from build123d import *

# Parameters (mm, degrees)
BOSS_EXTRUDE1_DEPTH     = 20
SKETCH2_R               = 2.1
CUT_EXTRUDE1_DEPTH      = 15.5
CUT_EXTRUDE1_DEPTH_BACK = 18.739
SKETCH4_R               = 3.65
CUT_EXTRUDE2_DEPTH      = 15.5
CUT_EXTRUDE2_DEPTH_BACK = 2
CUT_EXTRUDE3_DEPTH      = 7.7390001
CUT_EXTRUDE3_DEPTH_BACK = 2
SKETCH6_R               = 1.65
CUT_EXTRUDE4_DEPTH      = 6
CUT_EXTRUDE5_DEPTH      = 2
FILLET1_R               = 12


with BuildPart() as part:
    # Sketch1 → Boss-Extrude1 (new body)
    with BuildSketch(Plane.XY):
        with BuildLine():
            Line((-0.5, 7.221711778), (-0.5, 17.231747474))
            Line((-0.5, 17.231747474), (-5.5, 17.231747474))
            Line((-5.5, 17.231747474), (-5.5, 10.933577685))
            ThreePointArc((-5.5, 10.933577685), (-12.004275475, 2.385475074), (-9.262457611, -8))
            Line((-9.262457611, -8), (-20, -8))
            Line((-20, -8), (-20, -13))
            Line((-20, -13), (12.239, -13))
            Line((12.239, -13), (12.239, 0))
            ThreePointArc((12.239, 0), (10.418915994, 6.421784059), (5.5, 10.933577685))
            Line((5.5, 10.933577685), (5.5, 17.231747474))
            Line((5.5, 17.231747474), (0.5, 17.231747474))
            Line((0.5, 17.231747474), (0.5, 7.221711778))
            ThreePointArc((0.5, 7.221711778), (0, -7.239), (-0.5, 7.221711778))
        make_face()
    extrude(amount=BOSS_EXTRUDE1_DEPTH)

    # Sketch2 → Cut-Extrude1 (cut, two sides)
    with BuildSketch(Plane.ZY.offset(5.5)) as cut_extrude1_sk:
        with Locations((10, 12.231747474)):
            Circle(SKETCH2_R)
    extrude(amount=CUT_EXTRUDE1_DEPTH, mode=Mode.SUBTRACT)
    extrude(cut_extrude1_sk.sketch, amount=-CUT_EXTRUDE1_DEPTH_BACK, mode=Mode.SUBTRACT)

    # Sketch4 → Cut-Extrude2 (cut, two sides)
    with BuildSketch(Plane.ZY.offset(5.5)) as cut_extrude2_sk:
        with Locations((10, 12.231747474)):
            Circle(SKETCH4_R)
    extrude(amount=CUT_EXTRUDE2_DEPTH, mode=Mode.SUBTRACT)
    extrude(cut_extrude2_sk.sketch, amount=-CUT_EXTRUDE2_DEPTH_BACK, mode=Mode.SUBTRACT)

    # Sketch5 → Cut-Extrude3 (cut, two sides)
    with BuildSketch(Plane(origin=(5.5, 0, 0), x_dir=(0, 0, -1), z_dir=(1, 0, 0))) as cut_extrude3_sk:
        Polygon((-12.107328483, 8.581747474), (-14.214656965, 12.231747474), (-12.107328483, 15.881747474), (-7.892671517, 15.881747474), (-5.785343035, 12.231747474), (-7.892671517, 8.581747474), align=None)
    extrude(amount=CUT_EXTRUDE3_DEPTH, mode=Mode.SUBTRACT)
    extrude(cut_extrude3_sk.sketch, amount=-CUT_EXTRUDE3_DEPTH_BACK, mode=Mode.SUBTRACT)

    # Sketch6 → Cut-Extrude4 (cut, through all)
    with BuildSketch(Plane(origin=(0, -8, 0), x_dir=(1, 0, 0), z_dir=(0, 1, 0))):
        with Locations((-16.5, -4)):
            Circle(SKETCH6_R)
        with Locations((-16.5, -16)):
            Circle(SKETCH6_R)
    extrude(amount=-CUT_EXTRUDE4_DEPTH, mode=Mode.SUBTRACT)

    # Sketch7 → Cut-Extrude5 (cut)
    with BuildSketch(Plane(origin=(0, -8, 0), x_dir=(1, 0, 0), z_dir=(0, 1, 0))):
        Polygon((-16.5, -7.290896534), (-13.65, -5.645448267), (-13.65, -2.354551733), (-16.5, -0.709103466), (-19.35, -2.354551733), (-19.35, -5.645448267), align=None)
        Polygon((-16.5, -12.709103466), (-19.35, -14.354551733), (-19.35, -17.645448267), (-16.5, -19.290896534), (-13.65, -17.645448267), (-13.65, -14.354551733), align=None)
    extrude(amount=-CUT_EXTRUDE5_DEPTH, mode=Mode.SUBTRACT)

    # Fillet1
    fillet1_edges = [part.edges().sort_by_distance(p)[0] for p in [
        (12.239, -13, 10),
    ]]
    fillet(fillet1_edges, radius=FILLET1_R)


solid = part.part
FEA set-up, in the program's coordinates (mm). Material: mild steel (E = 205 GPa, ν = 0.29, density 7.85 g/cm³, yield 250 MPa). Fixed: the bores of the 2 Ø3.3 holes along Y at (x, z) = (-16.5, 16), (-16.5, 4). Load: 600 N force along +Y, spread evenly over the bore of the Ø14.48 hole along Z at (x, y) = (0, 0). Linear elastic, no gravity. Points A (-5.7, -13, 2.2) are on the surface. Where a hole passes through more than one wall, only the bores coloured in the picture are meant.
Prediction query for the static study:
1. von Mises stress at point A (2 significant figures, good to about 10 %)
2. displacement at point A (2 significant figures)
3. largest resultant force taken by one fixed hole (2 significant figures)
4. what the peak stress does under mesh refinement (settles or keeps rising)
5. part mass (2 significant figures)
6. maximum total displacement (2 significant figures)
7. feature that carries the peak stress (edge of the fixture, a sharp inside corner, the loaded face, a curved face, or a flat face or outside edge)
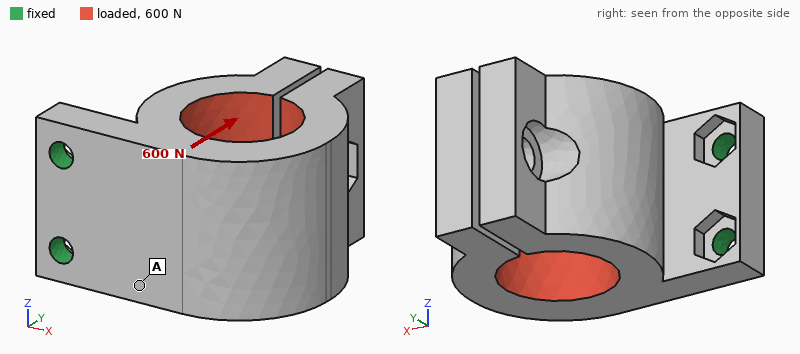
25 MPa
21 µm
300 N
keeps rising
65 g
89 µm
edge of the fixture
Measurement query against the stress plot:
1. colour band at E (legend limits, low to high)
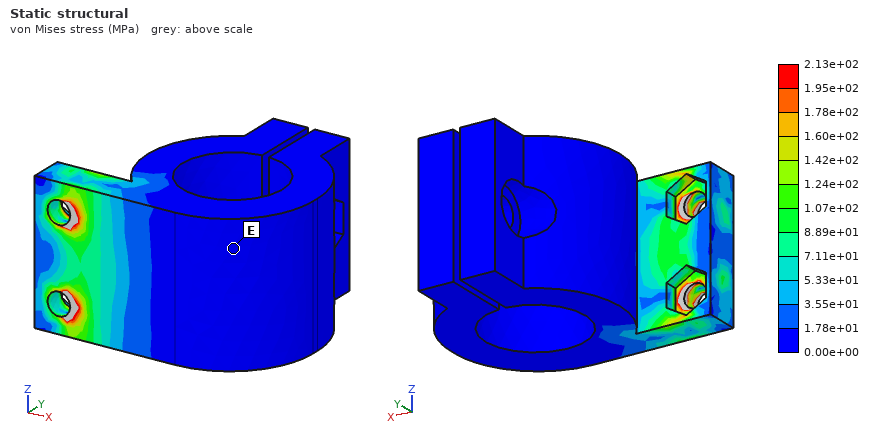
0.00e+00 to 1.78e+01 MPa
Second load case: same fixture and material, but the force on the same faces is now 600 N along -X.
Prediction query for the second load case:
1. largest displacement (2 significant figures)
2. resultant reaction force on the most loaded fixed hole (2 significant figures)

88 µm
300 N
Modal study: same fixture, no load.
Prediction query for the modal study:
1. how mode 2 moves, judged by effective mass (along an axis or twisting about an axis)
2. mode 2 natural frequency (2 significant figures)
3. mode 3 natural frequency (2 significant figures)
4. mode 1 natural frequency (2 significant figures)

along Z
3700 Hz
4700 Hz
1700 Hz
